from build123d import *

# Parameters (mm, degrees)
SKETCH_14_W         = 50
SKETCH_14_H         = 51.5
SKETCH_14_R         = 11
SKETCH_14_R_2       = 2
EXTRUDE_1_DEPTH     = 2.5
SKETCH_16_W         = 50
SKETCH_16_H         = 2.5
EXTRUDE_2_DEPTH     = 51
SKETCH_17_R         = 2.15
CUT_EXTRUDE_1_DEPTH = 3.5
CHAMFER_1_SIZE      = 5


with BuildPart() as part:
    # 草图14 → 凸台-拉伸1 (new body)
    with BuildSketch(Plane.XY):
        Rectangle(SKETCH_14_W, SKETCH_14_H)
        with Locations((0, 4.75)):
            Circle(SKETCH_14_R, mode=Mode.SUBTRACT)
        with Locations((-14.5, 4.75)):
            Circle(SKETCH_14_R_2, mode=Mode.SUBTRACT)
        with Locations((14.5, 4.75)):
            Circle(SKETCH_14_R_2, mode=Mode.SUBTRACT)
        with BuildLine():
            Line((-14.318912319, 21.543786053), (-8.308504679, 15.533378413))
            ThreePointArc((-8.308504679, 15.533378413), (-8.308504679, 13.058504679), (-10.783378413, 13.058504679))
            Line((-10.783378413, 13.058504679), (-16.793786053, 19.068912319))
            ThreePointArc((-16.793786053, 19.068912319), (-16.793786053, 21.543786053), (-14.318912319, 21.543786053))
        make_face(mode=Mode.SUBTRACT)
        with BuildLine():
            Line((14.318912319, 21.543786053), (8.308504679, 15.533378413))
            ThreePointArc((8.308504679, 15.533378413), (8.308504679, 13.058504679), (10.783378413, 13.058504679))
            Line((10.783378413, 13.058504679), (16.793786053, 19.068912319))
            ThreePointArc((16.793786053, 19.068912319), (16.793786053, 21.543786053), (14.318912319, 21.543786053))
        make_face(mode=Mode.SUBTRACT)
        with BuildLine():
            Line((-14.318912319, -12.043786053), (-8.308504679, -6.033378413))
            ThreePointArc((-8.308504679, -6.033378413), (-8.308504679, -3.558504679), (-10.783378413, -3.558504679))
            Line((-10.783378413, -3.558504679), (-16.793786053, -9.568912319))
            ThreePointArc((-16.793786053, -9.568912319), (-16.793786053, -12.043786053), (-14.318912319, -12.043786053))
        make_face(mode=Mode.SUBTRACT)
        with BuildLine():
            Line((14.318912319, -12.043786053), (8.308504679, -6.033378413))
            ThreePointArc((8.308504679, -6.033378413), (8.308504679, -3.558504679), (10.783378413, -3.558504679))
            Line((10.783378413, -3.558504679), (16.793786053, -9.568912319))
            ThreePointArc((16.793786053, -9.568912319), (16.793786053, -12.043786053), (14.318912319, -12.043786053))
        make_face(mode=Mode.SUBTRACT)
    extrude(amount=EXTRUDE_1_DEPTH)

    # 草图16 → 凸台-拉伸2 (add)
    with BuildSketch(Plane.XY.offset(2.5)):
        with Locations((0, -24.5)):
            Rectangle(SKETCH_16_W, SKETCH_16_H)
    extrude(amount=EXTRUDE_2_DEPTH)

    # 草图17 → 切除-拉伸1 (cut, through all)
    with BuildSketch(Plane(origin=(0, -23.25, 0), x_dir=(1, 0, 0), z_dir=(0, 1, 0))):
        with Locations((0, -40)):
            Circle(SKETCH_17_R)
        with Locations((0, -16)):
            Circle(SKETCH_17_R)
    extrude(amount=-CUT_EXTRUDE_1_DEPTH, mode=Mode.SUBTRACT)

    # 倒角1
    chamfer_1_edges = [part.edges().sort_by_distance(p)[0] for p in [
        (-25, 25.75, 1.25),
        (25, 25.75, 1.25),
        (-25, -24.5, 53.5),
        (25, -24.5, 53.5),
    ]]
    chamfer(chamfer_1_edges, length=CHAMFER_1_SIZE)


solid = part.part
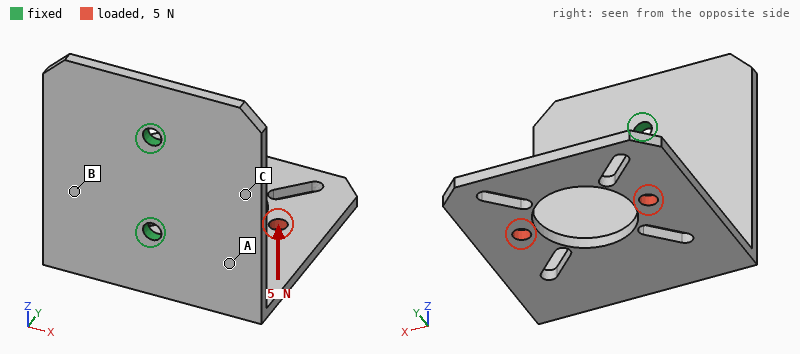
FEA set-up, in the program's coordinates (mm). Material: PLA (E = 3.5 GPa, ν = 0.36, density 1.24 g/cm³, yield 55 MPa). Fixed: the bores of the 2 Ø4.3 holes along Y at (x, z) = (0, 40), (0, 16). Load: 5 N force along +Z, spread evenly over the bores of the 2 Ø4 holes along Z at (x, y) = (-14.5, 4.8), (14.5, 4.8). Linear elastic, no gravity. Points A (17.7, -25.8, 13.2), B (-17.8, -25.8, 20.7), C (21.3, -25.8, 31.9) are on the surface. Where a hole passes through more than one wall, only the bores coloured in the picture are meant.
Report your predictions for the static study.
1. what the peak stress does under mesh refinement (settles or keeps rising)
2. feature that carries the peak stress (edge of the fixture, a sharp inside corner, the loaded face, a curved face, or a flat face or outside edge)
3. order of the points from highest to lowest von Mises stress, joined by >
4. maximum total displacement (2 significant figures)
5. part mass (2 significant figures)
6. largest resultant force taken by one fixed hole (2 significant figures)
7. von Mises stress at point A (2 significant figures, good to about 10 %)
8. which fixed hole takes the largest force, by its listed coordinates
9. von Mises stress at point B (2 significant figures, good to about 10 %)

keeps rising
edge of the fixture
A > B > C
0.96 mm
14 g
4.6 N
1.8 MPa
(0, 16)
1.1 MPa
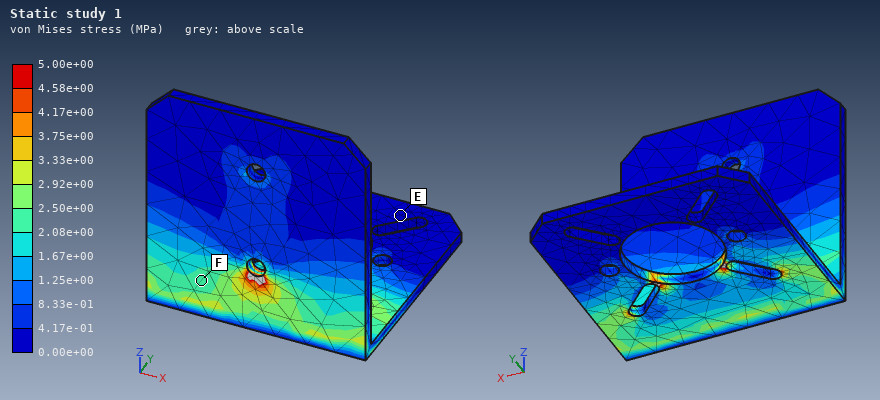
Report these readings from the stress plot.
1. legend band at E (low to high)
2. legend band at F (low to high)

0.00e+00 to 4.17e-01 MPa
2.08e+00 to 2.50e+00 MPa
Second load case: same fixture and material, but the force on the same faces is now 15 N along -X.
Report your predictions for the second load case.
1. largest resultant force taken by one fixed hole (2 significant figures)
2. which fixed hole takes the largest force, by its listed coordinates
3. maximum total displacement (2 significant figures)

23 N
(0, 16)
0.99 mm
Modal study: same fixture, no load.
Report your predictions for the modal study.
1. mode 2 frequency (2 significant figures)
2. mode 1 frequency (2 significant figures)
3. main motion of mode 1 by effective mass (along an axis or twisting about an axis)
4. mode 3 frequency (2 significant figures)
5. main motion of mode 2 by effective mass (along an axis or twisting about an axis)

300 Hz
190 Hz
along Z
500 Hz
along X
